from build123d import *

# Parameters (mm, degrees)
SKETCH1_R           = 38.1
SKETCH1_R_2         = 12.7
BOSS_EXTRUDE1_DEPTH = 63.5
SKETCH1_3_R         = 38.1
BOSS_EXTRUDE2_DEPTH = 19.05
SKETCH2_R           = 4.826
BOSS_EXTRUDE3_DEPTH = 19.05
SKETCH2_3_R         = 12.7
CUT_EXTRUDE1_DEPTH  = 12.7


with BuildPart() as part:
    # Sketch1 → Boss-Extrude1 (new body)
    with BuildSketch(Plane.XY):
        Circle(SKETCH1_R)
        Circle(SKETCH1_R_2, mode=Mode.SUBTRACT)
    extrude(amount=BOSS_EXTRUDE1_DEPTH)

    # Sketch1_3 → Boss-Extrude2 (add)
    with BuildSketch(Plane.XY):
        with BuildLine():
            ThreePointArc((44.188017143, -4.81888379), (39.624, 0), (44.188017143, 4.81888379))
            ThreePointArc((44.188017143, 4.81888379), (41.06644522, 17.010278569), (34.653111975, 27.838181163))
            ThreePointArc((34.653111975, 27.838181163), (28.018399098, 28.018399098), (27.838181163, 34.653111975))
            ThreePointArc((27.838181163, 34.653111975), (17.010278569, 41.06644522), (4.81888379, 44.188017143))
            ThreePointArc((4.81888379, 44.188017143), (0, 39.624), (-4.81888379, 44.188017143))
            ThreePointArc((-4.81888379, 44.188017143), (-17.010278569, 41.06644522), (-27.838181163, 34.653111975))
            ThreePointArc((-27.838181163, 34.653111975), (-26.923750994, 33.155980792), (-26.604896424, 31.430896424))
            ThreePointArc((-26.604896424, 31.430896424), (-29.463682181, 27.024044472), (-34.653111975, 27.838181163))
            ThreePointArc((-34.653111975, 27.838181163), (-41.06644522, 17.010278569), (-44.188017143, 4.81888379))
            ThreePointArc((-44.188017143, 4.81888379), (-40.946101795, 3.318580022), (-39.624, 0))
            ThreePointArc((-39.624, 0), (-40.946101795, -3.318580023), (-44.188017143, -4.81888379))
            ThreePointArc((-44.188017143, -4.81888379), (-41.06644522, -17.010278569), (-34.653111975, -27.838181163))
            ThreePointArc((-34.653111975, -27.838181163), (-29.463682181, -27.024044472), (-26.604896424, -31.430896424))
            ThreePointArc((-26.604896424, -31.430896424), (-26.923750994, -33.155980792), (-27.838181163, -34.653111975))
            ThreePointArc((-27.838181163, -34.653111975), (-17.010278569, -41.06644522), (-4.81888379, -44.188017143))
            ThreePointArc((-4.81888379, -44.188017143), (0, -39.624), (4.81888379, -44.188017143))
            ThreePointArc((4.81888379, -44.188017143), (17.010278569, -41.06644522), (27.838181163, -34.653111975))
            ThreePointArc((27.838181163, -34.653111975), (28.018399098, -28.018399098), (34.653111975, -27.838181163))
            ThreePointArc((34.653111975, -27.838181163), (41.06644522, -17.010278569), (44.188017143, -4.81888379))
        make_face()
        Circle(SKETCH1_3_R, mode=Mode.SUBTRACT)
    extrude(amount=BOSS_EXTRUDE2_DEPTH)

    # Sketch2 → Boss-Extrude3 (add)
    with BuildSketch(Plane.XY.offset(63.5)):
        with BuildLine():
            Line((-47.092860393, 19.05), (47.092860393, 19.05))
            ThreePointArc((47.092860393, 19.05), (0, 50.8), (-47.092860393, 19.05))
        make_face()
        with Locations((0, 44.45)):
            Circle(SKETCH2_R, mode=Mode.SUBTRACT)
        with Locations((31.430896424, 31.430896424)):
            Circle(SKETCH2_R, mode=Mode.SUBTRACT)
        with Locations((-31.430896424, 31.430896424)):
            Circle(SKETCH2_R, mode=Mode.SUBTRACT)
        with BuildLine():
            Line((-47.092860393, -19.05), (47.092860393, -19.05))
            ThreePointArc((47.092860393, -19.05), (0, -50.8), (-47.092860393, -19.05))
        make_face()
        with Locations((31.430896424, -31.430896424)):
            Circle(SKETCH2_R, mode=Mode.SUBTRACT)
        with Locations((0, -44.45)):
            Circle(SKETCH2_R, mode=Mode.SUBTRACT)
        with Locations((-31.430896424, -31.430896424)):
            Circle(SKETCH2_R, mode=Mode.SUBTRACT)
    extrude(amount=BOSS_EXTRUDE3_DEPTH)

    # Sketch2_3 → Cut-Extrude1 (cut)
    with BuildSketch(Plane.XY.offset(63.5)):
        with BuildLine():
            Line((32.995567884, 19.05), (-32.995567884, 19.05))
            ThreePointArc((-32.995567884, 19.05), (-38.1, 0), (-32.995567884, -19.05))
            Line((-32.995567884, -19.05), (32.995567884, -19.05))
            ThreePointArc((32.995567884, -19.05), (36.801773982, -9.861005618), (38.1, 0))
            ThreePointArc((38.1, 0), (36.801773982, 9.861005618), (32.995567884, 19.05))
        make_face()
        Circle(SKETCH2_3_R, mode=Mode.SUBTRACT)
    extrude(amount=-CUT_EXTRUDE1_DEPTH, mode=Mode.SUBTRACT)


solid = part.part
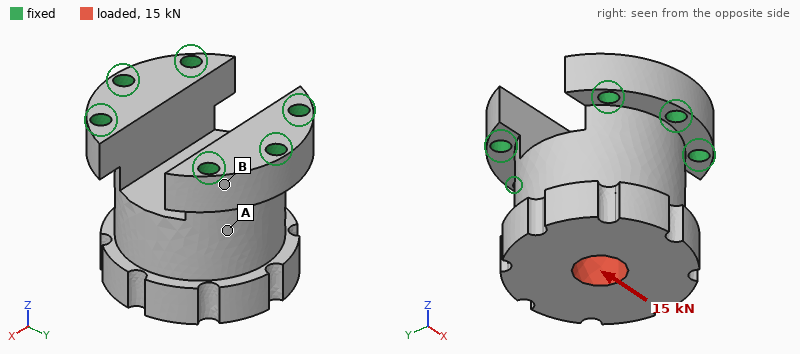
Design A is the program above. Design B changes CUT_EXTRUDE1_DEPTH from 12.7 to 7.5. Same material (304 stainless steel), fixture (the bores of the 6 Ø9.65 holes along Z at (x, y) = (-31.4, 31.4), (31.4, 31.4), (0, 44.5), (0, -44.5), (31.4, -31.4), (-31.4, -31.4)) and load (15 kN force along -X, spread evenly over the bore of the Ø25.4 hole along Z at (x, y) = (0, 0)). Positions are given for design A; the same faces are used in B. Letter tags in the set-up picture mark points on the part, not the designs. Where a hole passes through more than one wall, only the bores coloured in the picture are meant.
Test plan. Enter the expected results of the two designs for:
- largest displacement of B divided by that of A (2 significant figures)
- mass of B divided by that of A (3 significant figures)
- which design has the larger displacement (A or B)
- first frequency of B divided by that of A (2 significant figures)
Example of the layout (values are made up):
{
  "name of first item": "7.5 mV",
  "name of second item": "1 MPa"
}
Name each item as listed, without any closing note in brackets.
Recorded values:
{
  "largest displacement of B divided by that of A": "0.87",
  "mass of B divided by that of A": "1.04",
  "which design has the larger displacement": "A",
  "first frequency of B divided by that of A": "1.0"
}
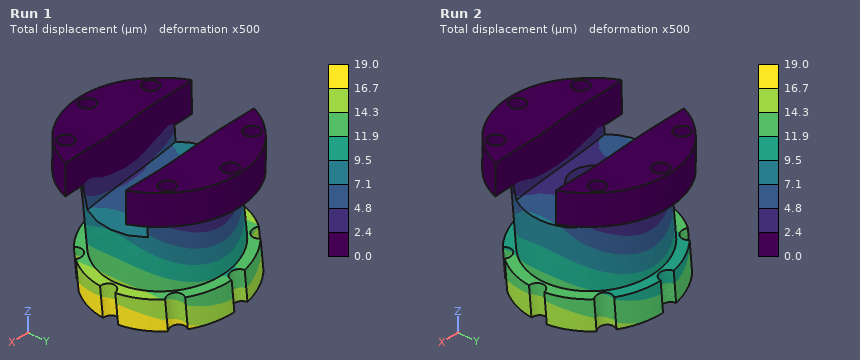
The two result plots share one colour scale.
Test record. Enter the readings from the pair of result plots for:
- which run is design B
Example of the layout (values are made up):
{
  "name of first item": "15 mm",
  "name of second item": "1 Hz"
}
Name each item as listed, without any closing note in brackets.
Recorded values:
{
  "which run is design B": "Run 2"
}
